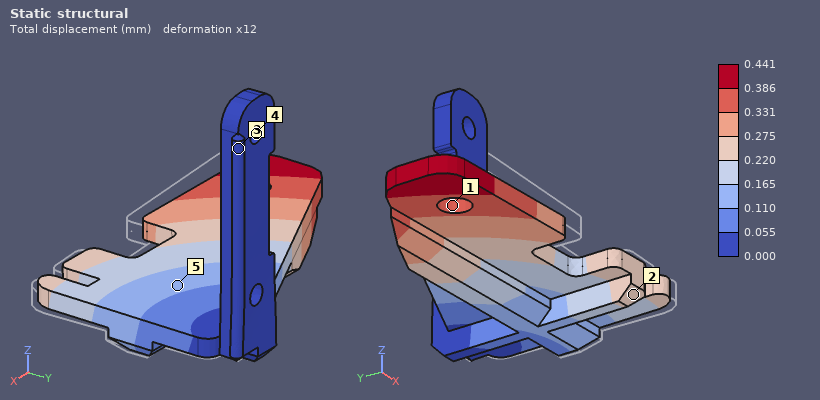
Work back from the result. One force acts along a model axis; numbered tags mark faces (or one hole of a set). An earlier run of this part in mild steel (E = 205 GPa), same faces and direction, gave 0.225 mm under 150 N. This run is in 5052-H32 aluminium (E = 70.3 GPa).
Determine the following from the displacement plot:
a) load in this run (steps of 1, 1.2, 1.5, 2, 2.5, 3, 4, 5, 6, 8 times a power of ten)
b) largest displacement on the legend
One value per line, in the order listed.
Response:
100 N
0.441 mm
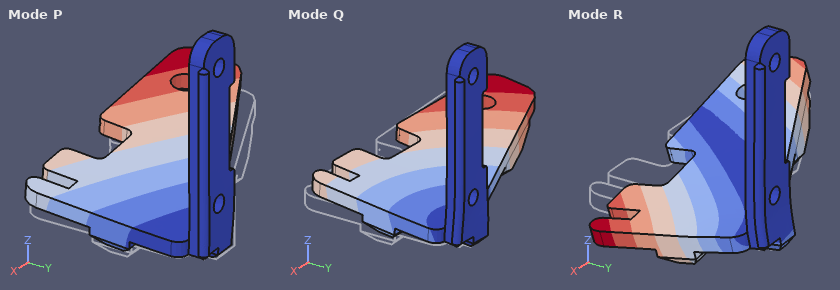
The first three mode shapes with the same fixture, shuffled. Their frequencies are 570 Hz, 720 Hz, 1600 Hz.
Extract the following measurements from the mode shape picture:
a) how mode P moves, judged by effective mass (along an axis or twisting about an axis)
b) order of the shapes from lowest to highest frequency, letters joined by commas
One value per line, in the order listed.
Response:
along Z
P, Q, R
